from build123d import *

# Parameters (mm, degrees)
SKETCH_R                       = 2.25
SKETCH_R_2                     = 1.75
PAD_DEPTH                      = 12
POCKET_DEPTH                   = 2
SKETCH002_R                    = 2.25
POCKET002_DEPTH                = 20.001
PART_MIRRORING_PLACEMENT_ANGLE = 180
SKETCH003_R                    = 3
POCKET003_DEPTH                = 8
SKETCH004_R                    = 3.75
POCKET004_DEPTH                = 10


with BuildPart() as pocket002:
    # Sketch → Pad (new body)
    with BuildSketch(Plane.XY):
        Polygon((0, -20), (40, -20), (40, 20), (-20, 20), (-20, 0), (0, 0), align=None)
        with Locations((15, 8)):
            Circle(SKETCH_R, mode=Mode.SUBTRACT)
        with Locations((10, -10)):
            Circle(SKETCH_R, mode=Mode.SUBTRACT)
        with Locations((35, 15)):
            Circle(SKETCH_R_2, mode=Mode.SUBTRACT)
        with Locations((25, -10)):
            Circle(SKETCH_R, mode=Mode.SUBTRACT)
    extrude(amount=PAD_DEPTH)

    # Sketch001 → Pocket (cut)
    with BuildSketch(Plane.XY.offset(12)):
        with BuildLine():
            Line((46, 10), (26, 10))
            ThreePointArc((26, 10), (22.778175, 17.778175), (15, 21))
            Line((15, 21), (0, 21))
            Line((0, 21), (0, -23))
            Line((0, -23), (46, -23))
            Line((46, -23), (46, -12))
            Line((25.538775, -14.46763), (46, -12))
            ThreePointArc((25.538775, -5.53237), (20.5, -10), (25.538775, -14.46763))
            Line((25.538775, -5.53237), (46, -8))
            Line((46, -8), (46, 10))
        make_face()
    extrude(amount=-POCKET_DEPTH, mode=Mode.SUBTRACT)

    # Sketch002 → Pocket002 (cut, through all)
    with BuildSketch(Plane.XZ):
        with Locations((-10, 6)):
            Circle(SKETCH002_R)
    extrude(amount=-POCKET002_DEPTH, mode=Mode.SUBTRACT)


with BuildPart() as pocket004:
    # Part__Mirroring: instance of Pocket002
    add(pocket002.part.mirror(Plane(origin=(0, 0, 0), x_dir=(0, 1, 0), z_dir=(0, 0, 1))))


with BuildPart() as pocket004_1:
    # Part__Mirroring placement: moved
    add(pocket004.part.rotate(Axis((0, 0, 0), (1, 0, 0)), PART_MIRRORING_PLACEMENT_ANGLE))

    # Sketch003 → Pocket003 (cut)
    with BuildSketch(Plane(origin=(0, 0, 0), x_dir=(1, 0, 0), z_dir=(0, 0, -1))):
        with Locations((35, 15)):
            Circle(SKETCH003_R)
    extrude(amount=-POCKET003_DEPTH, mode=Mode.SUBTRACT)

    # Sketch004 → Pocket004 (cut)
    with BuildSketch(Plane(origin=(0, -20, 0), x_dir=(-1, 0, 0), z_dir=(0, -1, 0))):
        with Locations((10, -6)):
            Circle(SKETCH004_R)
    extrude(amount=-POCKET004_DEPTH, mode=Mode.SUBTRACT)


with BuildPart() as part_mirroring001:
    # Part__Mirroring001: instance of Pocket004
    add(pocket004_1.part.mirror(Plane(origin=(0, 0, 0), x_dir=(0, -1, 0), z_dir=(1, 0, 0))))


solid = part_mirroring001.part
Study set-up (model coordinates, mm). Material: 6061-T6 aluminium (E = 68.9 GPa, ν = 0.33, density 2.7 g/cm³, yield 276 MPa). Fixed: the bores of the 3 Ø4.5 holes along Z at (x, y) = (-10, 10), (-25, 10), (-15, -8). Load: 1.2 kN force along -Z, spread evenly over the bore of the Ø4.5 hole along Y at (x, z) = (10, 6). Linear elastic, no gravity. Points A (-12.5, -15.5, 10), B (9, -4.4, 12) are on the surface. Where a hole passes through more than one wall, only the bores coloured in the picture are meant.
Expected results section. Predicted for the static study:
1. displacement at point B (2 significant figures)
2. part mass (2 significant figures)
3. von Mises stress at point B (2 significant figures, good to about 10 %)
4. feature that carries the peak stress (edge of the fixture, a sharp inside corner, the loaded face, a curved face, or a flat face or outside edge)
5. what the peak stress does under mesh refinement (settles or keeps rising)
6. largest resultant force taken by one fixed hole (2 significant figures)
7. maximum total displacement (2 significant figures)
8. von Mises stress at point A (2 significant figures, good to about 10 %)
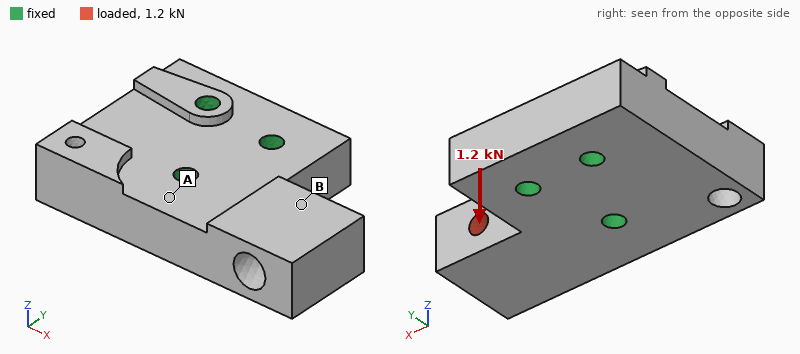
47 µm
54 g
8.7 MPa
edge of the fixture
keeps rising
760 N
75 µm
30 MPa
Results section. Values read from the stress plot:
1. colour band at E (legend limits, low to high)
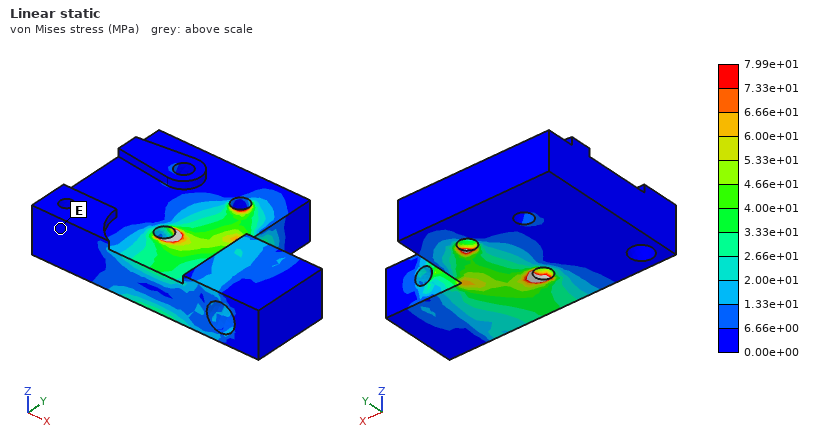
0.00e+00 to 6.66e+00 MPa
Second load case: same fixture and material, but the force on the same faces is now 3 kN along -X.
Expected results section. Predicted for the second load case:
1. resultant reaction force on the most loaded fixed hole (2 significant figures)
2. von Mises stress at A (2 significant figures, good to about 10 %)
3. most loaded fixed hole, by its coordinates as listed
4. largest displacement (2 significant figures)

2.3 kN
9.0 MPa
(-15, -8)
17 µm
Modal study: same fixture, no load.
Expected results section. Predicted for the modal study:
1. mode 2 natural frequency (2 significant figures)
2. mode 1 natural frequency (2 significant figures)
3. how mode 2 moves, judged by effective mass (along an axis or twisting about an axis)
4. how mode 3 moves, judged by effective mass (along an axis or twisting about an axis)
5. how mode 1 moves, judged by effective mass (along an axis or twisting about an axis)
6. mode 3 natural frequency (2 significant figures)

13 kHz
6800 Hz
along Y
along Z
along Z
15 kHz
